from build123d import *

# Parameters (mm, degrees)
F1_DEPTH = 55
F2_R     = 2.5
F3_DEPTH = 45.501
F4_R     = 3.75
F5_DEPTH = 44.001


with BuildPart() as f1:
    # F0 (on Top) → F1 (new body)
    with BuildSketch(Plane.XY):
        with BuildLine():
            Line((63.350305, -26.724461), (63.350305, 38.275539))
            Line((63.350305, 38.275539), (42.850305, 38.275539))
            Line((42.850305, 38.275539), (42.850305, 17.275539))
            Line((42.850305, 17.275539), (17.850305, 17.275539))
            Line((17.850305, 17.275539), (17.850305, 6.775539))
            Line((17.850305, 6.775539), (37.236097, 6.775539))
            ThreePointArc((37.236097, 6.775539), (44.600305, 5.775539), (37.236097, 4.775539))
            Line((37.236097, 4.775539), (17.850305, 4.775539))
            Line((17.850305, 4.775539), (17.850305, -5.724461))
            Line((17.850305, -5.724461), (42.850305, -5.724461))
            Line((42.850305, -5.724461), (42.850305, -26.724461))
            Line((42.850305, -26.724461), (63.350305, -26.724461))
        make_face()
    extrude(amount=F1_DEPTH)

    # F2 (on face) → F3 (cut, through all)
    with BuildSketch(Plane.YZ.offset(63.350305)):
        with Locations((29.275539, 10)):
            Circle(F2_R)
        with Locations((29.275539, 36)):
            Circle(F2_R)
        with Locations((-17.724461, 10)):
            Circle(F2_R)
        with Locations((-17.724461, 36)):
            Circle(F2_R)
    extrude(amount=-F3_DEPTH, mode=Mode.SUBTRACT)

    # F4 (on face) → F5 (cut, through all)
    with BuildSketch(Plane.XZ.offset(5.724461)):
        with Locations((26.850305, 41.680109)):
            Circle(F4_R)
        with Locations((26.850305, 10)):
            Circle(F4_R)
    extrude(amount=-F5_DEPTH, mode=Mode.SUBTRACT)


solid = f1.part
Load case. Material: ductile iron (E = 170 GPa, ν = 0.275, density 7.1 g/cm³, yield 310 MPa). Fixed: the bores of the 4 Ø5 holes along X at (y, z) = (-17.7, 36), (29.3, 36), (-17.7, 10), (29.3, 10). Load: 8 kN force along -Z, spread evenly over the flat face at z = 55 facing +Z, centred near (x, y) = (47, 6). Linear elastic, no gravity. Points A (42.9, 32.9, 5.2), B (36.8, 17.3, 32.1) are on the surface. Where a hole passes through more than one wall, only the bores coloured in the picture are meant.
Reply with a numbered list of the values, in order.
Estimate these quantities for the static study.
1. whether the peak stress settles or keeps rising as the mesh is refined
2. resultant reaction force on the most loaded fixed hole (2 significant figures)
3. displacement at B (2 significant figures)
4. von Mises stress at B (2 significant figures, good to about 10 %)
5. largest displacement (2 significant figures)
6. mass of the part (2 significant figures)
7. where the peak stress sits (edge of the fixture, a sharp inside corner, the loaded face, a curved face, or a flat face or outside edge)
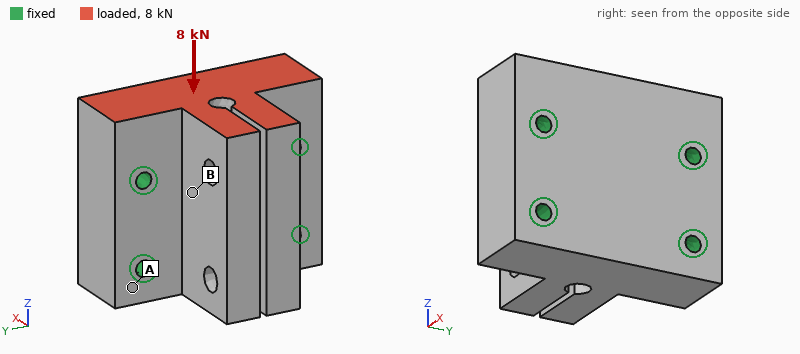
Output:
1. keeps rising
2. 2.9 kN
3. 1.6 µm
4. 5.6 MPa
5. 3.8 µm
6. 690 g
7. edge of the fixture
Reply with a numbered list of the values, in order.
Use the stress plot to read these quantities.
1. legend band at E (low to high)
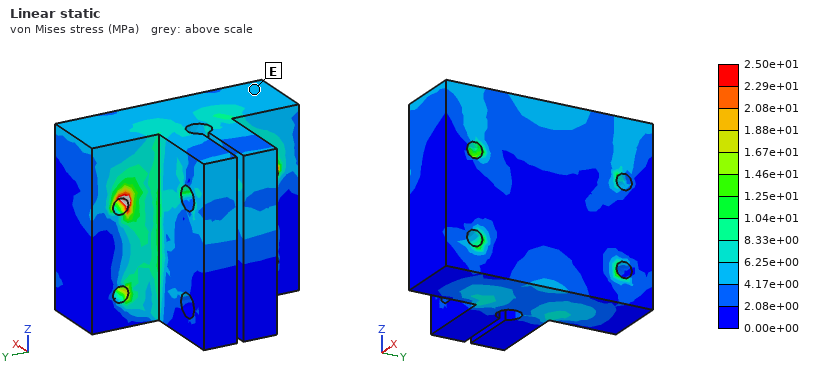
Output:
1. 4.17e+00 to 6.25e+00 MPa
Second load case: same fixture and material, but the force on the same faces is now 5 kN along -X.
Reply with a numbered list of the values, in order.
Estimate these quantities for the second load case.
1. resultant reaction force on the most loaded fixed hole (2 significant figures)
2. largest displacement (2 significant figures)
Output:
1. 3.0 kN
2. 6.6 µm
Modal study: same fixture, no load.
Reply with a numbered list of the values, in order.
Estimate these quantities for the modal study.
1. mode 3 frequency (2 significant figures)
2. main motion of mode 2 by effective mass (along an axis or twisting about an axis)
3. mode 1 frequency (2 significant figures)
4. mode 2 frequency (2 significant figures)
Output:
1. 11 kHz
2. along Y
3. 7100 Hz
4. 7400 Hz
